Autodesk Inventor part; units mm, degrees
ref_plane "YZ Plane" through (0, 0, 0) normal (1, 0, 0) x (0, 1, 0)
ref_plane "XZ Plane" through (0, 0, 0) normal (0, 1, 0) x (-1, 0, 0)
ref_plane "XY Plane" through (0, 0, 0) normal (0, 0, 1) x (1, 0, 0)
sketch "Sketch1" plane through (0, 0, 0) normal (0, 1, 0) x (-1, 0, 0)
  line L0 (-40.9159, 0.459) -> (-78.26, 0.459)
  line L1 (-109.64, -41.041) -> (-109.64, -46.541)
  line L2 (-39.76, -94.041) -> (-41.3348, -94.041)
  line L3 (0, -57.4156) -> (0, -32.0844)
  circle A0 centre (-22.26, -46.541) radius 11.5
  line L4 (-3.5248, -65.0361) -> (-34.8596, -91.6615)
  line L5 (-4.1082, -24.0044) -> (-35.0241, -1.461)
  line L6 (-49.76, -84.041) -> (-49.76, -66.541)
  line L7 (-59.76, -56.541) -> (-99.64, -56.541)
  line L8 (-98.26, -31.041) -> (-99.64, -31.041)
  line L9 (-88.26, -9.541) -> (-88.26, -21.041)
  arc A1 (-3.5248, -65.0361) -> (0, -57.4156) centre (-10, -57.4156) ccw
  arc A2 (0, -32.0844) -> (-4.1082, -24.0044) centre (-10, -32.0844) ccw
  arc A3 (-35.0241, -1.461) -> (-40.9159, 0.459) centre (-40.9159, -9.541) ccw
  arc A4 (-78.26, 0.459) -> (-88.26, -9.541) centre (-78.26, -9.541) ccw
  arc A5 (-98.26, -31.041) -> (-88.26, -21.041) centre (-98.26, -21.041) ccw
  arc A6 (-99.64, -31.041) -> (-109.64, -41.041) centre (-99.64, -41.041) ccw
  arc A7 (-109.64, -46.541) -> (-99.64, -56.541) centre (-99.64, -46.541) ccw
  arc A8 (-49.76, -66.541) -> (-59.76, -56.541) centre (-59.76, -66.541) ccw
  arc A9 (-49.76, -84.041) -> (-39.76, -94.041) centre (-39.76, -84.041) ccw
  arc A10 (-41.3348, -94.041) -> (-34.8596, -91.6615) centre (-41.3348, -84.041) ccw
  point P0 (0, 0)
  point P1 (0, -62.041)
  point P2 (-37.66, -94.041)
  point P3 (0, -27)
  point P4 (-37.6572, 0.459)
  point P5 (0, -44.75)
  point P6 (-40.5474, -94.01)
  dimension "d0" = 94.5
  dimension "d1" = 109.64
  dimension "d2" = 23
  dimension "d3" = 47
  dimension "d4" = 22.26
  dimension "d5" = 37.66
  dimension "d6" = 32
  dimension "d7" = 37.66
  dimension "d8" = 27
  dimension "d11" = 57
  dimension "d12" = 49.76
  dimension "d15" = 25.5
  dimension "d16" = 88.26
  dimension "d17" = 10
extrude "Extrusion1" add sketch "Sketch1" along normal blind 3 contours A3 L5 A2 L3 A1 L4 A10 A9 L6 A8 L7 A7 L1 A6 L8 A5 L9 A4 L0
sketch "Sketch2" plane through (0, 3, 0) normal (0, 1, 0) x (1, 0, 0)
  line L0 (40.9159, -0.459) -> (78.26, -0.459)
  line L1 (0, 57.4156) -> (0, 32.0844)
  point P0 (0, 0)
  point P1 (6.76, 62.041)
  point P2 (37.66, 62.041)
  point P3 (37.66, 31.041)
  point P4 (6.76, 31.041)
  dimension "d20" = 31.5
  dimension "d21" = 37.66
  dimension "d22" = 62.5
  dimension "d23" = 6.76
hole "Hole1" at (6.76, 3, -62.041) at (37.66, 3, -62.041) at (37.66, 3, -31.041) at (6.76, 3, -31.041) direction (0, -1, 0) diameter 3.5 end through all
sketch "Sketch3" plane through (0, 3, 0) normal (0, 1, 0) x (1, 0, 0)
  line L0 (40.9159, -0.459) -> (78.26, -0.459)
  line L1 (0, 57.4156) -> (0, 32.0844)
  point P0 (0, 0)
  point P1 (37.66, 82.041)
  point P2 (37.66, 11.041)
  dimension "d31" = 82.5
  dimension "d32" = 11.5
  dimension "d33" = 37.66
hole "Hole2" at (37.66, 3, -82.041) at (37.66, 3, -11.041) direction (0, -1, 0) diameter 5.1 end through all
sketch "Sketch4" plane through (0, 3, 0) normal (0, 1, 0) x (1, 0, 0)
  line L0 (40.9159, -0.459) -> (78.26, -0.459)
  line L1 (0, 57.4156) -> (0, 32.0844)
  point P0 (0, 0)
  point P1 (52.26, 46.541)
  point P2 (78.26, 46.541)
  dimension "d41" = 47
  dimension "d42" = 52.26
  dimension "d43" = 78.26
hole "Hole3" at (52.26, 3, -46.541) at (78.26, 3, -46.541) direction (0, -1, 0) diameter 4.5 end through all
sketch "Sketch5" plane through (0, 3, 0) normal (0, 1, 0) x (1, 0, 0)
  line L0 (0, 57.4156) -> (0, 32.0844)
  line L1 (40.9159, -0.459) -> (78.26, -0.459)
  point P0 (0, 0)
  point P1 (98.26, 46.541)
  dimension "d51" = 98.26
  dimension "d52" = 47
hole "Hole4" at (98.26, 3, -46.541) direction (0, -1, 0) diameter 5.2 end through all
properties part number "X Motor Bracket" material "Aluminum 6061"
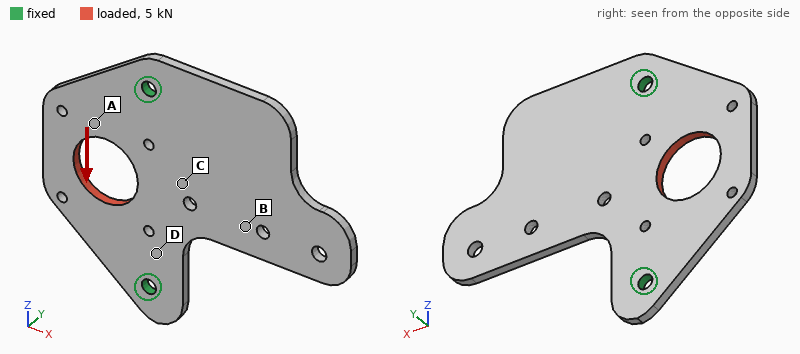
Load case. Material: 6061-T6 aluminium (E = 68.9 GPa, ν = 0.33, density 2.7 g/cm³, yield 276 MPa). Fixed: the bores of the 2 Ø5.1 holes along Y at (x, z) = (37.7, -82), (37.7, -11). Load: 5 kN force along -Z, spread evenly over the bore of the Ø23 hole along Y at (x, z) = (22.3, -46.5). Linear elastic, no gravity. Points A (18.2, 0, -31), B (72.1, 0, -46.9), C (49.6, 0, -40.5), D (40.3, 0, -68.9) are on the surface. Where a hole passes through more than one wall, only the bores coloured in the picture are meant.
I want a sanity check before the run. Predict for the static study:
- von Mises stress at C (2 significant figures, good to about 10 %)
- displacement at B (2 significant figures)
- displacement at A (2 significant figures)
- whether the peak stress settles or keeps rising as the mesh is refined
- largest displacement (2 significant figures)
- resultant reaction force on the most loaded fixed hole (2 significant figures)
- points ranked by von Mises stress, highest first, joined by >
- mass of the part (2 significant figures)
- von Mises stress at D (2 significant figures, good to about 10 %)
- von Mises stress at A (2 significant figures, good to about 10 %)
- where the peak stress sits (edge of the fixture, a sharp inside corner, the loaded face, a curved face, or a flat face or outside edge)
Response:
13 MPa
6.4 µm
28 µm
keeps rising
41 µm
2.8 kN
A > D > C > B
46 g
23 MPa
46 MPa
edge of the fixture
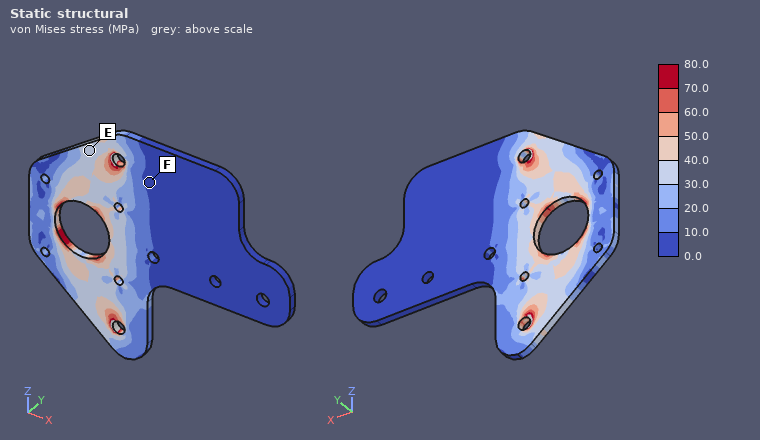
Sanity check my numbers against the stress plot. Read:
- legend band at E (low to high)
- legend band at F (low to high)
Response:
30.0 to 40.0 MPa
0.0 to 10.0 MPa
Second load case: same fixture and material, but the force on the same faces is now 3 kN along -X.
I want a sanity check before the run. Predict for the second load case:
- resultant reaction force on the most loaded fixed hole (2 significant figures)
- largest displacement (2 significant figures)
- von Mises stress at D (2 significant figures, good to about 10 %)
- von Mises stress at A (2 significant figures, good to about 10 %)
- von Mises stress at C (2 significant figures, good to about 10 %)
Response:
1.5 kN
38 µm
24 MPa
27 MPa
15 MPa
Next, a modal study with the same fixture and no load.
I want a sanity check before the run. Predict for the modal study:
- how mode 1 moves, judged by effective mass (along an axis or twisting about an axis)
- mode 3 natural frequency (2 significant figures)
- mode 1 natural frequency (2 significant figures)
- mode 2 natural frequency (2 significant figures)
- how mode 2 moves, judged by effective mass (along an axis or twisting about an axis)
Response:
along Y
1900 Hz
560 Hz
1600 Hz
along Y
